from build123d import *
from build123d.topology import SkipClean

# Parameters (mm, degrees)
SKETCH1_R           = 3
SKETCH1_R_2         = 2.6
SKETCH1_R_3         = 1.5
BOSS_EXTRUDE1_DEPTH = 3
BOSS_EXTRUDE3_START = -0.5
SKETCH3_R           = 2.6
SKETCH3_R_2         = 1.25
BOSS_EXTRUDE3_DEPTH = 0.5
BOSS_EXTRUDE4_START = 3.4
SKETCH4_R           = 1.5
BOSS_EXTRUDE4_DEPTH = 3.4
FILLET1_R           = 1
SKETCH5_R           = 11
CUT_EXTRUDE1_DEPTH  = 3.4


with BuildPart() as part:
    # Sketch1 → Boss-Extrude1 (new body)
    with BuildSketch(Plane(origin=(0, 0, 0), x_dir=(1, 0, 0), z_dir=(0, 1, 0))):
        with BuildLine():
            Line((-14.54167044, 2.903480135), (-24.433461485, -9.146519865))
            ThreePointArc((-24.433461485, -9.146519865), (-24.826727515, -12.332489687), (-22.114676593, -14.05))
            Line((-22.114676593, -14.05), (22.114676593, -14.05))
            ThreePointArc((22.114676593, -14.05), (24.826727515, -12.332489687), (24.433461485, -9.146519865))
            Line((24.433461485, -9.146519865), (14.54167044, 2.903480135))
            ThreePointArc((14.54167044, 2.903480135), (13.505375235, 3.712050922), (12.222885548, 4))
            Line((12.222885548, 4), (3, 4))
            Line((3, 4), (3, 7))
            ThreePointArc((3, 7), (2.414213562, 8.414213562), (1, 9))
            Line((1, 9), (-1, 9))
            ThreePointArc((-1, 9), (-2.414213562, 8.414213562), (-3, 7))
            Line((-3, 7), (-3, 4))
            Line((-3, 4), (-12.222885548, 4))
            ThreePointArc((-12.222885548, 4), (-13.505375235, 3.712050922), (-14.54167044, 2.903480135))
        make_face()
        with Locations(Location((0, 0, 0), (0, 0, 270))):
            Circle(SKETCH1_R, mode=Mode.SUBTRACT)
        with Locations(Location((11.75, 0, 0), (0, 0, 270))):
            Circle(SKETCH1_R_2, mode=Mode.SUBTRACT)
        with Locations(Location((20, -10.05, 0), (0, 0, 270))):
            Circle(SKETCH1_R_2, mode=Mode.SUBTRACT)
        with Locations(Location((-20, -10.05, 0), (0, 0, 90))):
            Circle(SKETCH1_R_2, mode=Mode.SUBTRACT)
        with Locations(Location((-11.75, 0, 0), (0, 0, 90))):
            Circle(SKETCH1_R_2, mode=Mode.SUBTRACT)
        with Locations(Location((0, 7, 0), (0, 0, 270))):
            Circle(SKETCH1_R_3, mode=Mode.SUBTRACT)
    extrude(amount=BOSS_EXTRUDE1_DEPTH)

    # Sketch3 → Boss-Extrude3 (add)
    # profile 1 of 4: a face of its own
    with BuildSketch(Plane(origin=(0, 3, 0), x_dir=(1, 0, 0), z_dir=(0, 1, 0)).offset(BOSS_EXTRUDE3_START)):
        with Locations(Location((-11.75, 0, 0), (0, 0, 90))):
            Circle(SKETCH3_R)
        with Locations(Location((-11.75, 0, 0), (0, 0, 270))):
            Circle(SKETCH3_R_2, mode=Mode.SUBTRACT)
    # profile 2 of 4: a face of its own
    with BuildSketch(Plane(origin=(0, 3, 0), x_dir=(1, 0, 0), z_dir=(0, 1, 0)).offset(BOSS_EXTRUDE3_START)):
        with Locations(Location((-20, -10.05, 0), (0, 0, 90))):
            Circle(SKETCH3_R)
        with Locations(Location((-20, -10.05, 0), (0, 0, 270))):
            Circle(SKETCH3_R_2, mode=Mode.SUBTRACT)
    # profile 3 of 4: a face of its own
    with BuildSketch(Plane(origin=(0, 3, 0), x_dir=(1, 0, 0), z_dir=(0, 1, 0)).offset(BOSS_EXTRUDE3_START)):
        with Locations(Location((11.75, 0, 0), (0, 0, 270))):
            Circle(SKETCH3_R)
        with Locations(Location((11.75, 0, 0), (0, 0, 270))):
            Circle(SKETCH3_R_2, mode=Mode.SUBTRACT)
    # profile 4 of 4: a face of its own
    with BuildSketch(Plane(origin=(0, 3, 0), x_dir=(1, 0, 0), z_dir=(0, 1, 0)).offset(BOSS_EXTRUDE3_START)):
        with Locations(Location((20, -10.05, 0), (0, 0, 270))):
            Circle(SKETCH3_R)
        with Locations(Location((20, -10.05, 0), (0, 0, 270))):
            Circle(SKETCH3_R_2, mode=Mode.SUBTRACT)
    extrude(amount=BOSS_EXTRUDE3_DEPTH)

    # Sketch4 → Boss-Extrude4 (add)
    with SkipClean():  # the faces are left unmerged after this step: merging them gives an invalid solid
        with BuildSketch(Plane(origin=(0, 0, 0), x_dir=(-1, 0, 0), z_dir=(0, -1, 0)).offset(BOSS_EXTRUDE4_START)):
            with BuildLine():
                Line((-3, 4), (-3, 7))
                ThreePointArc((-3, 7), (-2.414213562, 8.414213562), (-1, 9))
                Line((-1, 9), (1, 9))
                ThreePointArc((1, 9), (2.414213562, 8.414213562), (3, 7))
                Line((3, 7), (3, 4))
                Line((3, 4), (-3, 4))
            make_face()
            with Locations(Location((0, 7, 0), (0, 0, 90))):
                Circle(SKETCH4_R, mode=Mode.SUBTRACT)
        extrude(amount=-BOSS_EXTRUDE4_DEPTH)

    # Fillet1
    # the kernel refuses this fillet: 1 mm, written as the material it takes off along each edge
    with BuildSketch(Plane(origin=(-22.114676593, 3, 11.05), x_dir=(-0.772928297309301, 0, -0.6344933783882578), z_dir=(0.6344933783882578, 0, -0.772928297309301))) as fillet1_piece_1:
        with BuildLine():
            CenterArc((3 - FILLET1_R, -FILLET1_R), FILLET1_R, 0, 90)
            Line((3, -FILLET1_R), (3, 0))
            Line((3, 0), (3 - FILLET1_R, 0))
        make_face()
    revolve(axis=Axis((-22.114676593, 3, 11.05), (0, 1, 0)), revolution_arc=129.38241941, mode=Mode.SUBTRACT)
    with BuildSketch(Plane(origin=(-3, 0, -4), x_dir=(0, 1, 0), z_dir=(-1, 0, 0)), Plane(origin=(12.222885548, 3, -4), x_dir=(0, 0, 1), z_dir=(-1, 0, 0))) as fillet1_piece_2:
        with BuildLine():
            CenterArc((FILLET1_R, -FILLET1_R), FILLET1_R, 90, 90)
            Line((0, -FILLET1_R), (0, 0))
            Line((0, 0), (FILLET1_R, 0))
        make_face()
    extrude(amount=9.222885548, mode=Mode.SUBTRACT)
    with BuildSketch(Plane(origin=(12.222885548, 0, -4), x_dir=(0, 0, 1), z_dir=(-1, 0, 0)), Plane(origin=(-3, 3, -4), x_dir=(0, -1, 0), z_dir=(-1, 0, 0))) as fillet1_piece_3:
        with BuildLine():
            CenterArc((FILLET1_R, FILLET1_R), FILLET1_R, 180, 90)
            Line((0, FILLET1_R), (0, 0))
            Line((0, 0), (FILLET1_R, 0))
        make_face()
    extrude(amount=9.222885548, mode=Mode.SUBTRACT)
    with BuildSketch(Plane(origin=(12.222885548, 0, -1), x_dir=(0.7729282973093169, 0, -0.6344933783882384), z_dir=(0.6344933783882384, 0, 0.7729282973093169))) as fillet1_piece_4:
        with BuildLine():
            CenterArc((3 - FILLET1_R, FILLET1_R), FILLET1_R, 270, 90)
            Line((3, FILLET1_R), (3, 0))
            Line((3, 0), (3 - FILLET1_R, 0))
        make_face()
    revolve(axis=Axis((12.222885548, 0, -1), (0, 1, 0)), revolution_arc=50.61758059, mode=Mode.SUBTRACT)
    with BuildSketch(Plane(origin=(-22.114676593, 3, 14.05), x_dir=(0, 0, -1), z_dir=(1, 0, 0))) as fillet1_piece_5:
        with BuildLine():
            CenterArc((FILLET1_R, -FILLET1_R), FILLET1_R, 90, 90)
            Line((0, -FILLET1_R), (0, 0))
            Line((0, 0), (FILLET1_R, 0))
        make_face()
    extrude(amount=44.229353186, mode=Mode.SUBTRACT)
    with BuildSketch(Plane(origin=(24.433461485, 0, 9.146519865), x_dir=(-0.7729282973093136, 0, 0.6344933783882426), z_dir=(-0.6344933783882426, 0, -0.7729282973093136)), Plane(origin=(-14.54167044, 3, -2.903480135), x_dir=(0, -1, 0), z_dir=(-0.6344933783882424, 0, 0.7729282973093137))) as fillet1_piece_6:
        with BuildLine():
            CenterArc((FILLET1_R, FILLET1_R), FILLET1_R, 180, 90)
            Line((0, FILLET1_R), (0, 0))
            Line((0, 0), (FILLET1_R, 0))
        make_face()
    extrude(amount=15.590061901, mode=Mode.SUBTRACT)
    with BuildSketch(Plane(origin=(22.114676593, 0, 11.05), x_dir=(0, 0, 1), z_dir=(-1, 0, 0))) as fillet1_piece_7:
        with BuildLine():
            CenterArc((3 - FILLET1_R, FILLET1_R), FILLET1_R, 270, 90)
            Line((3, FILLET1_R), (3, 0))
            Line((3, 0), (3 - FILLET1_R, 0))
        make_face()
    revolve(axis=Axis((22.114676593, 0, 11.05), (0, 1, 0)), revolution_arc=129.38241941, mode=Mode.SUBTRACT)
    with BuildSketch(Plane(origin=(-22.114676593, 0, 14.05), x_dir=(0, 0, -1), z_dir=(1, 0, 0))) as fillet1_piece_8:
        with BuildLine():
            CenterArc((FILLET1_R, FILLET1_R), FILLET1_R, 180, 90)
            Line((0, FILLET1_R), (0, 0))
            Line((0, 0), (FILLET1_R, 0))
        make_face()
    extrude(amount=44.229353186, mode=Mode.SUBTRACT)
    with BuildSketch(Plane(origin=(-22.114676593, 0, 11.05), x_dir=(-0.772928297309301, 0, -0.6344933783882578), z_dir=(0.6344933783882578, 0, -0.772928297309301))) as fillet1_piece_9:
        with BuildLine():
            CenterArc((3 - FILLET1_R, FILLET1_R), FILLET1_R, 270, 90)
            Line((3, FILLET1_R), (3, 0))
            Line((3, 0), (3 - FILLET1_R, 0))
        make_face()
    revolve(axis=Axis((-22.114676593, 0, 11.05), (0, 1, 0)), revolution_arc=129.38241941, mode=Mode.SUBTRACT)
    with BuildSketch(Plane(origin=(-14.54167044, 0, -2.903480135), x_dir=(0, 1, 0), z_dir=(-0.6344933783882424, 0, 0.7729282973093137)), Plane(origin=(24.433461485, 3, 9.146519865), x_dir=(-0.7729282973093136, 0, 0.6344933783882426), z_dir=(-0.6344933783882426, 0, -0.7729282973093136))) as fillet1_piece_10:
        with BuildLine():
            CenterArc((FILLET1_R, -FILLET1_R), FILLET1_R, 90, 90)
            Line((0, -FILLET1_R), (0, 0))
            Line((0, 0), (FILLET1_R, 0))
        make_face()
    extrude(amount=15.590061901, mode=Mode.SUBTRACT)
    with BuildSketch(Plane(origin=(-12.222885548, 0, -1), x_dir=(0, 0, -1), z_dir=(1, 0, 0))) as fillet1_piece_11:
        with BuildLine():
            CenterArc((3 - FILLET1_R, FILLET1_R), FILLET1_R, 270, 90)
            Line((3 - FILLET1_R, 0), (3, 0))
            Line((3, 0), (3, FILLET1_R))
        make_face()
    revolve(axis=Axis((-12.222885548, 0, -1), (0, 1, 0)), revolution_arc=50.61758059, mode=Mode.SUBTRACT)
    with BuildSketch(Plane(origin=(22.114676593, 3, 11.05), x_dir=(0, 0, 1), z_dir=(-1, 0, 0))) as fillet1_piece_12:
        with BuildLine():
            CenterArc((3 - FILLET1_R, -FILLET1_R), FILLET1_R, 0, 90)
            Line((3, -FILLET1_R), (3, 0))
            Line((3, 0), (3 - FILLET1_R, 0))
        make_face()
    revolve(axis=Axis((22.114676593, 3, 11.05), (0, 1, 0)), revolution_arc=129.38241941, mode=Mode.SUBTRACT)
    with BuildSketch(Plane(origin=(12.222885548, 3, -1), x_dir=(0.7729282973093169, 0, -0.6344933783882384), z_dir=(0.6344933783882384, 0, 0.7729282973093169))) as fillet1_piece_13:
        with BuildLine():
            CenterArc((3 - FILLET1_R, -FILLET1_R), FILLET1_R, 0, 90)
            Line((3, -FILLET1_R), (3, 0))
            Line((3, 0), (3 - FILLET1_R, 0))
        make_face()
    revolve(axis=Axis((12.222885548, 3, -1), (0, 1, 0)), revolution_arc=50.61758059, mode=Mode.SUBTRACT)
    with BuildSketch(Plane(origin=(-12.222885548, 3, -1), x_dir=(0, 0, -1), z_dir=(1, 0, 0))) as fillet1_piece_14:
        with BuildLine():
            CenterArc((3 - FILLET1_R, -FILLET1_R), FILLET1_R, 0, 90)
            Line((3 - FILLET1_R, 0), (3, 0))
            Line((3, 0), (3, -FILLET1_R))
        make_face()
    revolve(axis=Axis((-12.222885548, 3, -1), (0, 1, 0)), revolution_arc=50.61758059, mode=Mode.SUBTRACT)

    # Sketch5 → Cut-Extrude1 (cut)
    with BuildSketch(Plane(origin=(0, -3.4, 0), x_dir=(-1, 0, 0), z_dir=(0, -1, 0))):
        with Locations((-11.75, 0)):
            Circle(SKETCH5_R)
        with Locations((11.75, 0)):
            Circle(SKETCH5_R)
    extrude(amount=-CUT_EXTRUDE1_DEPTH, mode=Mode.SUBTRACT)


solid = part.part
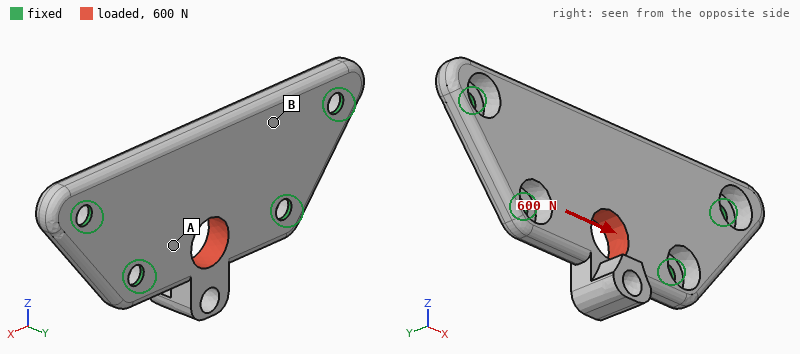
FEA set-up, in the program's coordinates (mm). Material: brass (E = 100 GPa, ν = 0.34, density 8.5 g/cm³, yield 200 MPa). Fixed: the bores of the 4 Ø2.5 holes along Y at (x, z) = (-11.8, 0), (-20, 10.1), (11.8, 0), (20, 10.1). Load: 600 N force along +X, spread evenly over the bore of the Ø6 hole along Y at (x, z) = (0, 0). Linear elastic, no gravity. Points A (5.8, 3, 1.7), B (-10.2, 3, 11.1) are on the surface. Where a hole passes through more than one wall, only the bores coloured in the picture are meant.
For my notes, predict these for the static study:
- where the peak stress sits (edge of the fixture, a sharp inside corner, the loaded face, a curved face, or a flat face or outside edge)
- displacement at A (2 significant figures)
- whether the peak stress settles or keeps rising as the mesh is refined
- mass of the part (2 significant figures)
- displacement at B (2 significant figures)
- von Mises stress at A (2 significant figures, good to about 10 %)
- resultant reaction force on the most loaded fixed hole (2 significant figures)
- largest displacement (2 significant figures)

edge of the fixture
1.8 µm
keeps rising
17 g
1.4 µm
16 MPa
210 N
3.2 µm
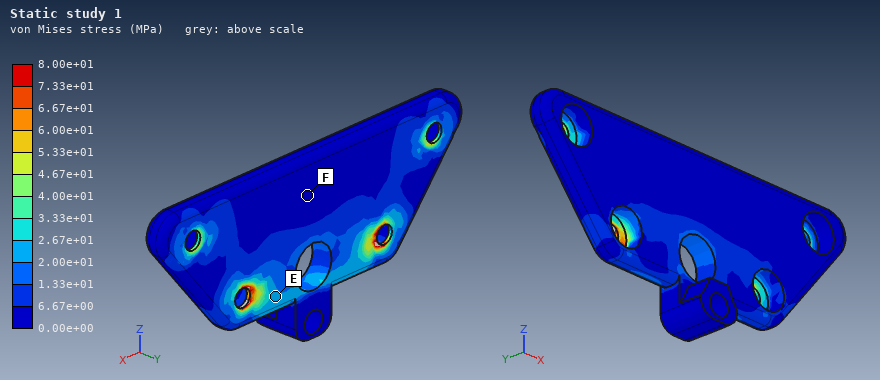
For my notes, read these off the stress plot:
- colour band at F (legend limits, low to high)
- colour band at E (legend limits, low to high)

0.00e+00 to 6.67e+00 MPa
2.00e+01 to 2.67e+01 MPa
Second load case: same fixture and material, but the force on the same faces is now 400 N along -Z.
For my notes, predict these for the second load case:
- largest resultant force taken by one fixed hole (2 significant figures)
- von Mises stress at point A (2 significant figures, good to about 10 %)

170 N
10 MPa
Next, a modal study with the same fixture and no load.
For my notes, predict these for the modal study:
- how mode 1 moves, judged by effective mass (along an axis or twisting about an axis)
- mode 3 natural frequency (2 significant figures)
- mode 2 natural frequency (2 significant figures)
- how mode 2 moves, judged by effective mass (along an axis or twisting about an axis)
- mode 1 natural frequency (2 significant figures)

along Y
13 kHz
7900 Hz
along Y
5300 Hz
